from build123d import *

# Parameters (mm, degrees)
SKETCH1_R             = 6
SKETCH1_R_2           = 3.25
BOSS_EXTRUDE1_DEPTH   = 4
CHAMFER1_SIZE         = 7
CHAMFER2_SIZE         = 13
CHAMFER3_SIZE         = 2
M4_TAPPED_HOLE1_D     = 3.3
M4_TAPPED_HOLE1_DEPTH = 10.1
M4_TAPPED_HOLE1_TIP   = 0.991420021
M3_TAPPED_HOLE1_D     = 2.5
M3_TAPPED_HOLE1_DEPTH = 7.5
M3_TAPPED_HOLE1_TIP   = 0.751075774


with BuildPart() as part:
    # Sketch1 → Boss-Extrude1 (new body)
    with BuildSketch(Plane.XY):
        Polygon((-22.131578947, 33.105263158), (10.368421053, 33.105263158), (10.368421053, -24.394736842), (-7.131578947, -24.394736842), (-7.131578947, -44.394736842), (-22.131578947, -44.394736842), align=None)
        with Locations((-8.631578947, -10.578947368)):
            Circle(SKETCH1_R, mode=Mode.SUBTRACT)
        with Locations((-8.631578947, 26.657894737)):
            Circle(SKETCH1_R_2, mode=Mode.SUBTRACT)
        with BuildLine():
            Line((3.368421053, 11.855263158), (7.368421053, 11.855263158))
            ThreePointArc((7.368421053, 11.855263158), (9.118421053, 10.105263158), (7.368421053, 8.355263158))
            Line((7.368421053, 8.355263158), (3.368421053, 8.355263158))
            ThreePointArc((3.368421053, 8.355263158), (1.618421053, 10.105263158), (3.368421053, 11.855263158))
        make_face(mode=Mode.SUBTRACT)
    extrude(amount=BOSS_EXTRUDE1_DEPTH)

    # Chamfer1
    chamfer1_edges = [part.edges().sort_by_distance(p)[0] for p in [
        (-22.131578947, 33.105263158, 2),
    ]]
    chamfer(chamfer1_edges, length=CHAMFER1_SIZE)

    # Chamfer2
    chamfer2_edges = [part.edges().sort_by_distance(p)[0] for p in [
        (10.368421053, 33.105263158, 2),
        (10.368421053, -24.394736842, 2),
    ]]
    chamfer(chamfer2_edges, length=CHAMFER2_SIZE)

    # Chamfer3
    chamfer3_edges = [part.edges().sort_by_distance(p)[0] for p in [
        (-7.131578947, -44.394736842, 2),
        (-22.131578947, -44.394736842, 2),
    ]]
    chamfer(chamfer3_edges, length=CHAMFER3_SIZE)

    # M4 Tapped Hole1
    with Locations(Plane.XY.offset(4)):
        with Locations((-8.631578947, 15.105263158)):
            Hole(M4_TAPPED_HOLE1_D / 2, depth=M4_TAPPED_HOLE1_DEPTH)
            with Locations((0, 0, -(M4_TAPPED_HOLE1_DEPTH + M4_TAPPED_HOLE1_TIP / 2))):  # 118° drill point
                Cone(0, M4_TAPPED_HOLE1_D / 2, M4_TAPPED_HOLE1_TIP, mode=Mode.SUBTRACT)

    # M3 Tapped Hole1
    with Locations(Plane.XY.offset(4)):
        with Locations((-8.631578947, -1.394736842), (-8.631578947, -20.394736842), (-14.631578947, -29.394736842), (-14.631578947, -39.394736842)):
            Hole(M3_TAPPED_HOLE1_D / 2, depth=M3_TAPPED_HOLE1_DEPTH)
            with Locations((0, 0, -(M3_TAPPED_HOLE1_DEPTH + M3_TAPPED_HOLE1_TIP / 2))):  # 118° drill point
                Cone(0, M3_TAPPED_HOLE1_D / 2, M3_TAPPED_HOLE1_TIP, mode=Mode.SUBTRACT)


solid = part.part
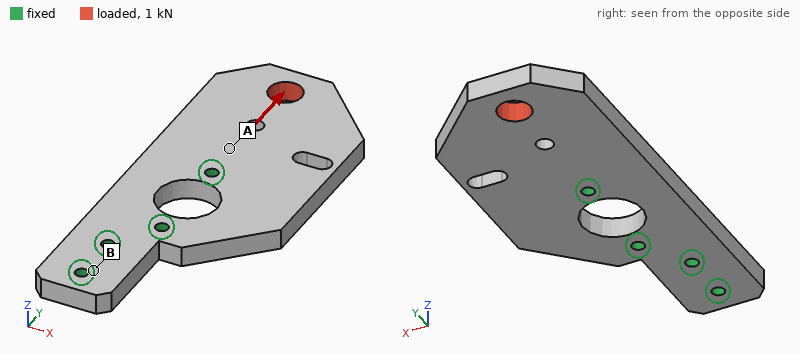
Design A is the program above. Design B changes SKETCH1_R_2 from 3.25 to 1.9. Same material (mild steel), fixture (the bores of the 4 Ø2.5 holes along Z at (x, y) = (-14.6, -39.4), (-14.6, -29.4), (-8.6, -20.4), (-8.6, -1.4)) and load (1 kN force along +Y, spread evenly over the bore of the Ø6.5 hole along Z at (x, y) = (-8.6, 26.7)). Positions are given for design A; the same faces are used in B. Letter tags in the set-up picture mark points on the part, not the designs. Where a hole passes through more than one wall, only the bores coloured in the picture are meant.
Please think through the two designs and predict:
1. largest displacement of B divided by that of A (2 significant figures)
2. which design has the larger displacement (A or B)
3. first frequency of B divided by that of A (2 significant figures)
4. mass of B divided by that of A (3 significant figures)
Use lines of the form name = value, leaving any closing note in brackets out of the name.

largest displacement of B divided by that of A = 0.92
which design has the larger displacement = A
first frequency of B divided by that of A = 0.97
mass of B divided by that of A = 1.01
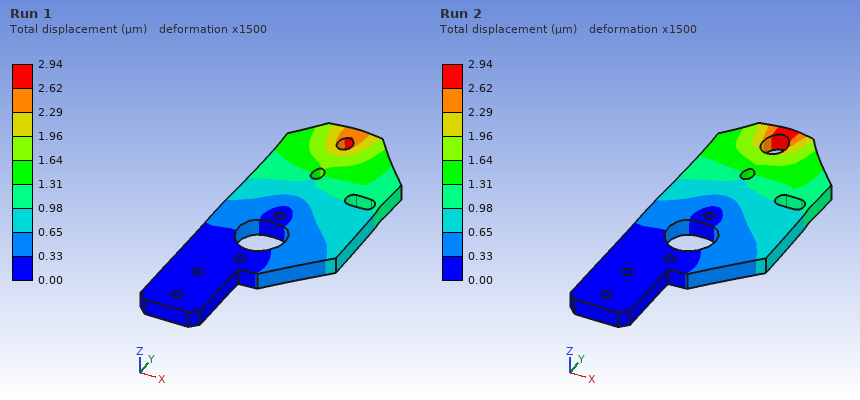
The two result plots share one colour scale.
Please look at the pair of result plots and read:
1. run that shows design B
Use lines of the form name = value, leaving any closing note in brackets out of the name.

run that shows design B = Run 1
